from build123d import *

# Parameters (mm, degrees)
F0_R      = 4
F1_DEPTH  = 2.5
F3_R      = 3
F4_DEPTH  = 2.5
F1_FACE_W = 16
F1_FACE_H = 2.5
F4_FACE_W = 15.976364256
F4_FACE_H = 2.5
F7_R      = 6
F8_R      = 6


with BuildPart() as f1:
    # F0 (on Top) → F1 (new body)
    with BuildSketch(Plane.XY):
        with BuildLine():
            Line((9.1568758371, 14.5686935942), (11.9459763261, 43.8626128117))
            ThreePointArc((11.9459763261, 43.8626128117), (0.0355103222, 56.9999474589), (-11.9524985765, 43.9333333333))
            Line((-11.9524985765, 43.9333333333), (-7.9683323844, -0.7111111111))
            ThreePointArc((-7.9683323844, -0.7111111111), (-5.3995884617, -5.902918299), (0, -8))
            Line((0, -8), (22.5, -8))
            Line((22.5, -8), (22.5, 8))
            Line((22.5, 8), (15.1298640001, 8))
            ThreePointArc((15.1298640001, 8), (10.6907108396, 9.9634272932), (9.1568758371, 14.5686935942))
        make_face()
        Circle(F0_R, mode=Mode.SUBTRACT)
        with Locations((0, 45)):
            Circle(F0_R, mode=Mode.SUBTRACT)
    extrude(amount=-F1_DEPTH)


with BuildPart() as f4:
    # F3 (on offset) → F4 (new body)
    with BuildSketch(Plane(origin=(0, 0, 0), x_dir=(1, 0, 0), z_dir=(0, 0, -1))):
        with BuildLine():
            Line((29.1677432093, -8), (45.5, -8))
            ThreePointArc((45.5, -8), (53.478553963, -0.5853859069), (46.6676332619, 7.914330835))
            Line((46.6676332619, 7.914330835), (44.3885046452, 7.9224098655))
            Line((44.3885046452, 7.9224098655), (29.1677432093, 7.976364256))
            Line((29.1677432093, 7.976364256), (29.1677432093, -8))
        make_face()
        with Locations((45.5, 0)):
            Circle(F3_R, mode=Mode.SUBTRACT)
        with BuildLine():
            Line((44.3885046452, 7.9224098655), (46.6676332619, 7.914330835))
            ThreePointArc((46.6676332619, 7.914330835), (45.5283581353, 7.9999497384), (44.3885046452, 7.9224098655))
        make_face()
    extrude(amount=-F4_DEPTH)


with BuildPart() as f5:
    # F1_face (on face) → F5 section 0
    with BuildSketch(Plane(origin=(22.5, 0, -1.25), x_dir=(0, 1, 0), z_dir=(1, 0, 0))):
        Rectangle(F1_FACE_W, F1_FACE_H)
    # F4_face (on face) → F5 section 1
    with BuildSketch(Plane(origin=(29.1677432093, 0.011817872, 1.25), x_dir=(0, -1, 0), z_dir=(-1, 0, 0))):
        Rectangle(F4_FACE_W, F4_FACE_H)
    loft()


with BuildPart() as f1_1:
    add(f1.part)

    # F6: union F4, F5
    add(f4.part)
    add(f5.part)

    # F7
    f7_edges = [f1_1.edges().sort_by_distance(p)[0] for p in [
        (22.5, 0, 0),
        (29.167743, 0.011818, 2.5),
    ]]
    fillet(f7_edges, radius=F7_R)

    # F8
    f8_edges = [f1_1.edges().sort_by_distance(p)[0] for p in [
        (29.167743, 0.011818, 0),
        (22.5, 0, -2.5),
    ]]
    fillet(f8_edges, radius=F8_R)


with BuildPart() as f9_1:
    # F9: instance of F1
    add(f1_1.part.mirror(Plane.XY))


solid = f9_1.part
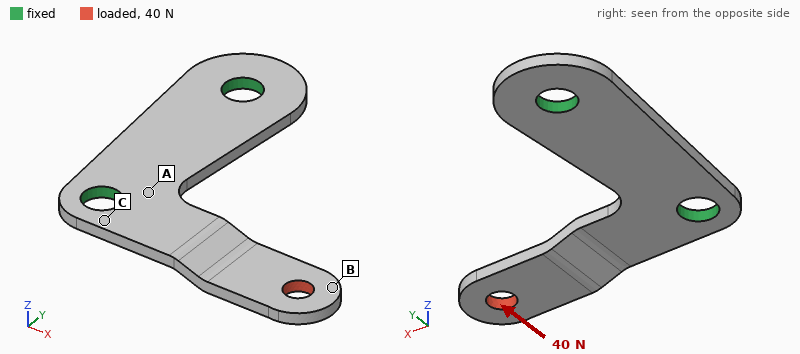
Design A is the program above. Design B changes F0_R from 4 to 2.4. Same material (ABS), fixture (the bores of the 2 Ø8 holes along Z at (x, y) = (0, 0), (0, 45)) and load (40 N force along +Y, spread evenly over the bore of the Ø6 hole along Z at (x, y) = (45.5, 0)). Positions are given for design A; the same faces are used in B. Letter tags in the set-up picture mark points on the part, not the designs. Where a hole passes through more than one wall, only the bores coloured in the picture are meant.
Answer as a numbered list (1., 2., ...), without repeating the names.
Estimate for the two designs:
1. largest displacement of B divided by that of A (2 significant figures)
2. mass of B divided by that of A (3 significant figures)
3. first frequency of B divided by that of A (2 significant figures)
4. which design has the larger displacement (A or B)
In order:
1. 1.1
2. 1.04
3. 0.94
4. B
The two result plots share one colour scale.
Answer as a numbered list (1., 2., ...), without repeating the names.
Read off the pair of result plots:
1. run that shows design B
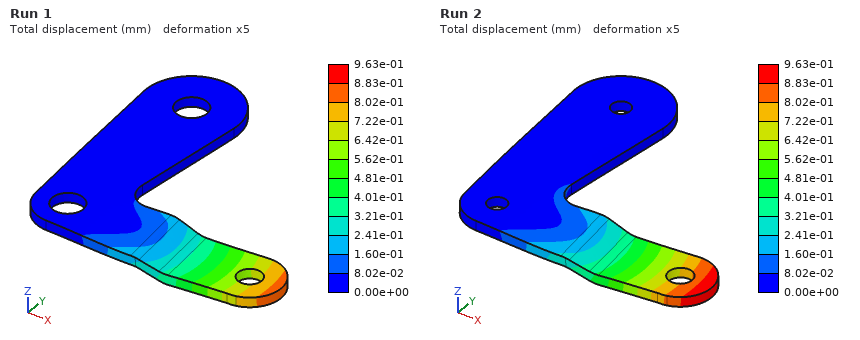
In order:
1. Run 2
